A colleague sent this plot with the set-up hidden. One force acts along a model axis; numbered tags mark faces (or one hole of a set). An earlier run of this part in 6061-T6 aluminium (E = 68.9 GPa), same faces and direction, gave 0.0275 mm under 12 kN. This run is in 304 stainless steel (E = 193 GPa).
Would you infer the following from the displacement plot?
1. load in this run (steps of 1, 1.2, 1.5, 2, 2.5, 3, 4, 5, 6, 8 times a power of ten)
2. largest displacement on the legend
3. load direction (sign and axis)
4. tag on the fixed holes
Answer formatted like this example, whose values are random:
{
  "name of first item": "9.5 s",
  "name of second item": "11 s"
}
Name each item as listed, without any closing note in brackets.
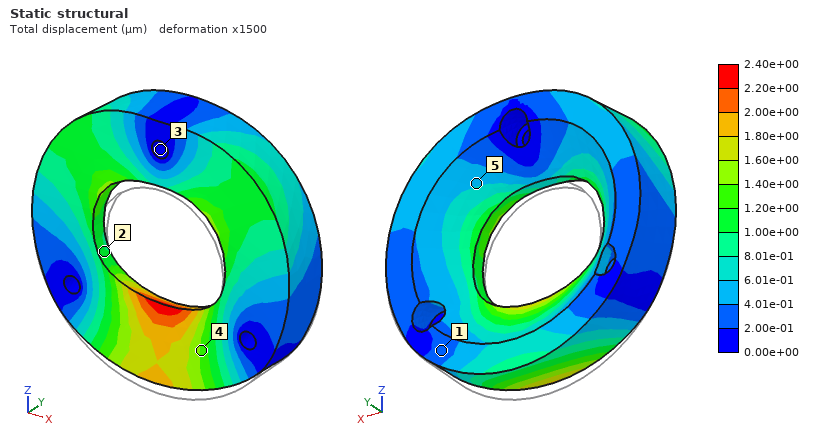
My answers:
{
  "load in this run": "3 kN",
  "largest displacement on the legend": "2.40e+00 µm",
  "load direction": "+Z",
  "tag on the fixed holes": "3"
}
